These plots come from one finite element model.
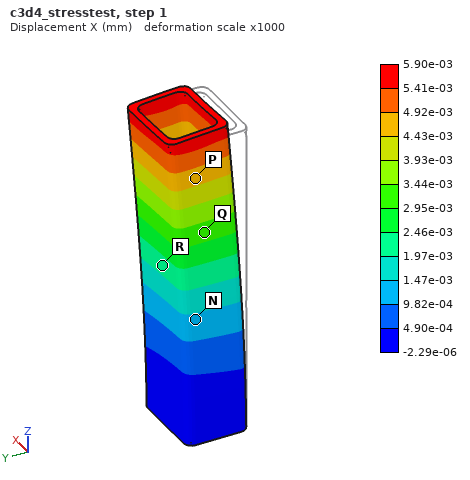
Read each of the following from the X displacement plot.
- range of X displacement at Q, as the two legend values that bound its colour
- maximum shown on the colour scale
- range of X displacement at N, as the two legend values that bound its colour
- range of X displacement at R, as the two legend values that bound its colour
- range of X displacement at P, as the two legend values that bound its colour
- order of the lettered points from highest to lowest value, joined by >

2.95e-03 to 3.44e-03 mm
5.90e-03 mm
9.82e-04 to 1.47e-03 mm
1.97e-03 to 2.46e-03 mm
4.43e-03 to 4.92e-03 mm
P > Q > R > N
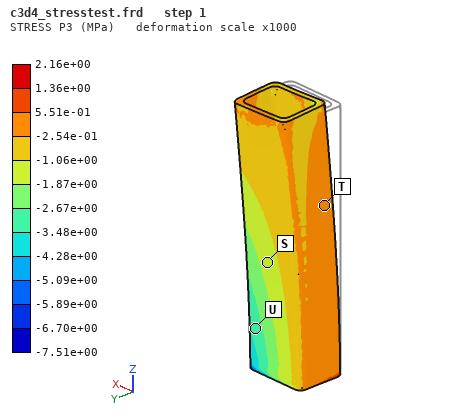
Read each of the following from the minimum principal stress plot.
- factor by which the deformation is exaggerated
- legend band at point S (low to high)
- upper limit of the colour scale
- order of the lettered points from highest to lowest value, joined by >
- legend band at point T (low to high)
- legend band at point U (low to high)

1000
-1.87e+00 to -1.06e+00 MPa
2.16e+00 MPa
T > S > U
-2.54e-01 to 5.51e-01 MPa
-3.48e+00 to -2.67e+00 MPa
